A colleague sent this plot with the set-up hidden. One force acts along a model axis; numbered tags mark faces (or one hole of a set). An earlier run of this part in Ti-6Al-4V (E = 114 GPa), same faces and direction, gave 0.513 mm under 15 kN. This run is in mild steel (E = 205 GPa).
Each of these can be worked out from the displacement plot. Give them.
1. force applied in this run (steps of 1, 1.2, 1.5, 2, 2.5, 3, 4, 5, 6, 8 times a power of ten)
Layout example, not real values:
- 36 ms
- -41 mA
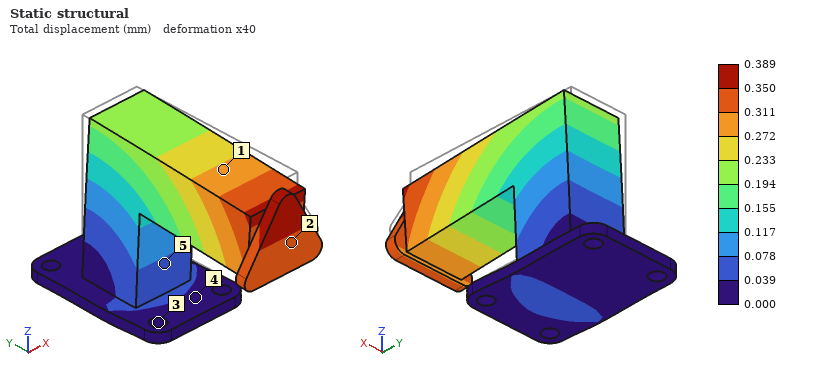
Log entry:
- 20 kN
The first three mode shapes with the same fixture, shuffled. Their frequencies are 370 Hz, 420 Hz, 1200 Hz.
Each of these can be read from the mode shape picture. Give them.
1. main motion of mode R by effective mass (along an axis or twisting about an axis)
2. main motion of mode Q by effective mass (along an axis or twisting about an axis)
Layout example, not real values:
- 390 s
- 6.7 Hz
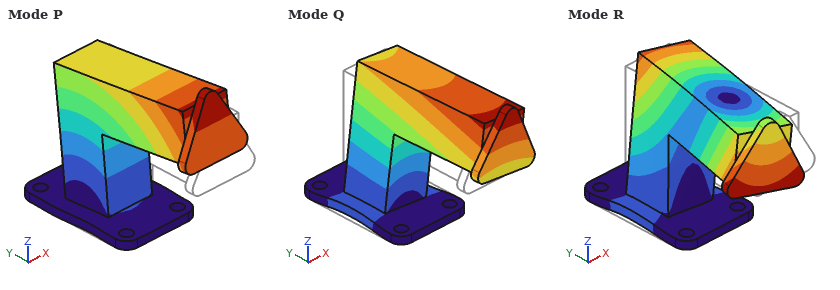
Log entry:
- twisting about Z
- along X
